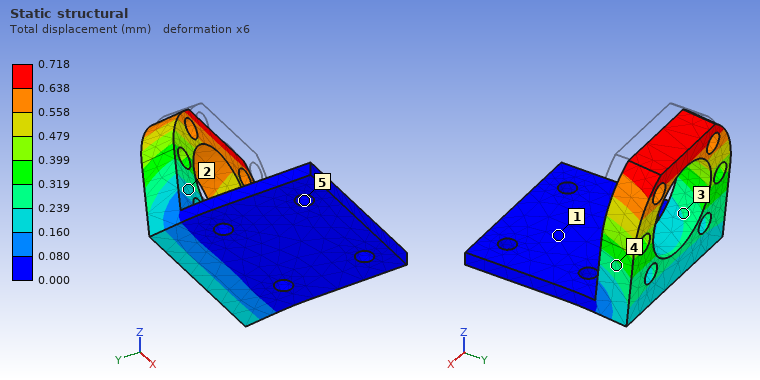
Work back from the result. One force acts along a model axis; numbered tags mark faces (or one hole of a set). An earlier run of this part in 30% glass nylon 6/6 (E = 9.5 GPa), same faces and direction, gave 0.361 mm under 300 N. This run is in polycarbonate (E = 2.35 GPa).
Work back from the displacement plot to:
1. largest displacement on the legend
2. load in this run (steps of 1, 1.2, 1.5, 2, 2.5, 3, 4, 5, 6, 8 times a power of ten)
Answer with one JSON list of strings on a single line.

["0.718 mm", "150 N"]
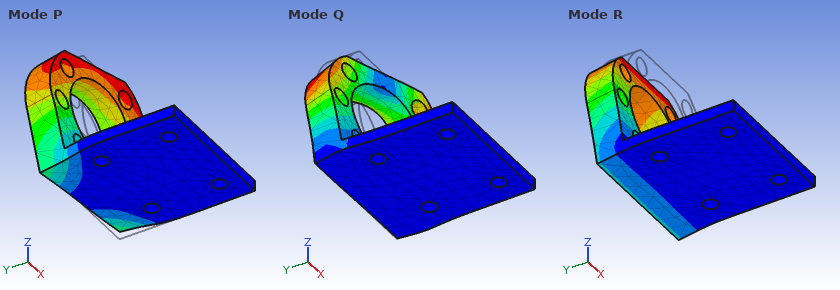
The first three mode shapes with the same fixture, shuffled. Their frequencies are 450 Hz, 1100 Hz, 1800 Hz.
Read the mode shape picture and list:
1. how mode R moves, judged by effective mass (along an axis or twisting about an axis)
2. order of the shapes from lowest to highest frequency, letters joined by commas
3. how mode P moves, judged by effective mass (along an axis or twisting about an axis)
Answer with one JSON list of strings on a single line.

["along Y", "R, P, Q", "along X"]
